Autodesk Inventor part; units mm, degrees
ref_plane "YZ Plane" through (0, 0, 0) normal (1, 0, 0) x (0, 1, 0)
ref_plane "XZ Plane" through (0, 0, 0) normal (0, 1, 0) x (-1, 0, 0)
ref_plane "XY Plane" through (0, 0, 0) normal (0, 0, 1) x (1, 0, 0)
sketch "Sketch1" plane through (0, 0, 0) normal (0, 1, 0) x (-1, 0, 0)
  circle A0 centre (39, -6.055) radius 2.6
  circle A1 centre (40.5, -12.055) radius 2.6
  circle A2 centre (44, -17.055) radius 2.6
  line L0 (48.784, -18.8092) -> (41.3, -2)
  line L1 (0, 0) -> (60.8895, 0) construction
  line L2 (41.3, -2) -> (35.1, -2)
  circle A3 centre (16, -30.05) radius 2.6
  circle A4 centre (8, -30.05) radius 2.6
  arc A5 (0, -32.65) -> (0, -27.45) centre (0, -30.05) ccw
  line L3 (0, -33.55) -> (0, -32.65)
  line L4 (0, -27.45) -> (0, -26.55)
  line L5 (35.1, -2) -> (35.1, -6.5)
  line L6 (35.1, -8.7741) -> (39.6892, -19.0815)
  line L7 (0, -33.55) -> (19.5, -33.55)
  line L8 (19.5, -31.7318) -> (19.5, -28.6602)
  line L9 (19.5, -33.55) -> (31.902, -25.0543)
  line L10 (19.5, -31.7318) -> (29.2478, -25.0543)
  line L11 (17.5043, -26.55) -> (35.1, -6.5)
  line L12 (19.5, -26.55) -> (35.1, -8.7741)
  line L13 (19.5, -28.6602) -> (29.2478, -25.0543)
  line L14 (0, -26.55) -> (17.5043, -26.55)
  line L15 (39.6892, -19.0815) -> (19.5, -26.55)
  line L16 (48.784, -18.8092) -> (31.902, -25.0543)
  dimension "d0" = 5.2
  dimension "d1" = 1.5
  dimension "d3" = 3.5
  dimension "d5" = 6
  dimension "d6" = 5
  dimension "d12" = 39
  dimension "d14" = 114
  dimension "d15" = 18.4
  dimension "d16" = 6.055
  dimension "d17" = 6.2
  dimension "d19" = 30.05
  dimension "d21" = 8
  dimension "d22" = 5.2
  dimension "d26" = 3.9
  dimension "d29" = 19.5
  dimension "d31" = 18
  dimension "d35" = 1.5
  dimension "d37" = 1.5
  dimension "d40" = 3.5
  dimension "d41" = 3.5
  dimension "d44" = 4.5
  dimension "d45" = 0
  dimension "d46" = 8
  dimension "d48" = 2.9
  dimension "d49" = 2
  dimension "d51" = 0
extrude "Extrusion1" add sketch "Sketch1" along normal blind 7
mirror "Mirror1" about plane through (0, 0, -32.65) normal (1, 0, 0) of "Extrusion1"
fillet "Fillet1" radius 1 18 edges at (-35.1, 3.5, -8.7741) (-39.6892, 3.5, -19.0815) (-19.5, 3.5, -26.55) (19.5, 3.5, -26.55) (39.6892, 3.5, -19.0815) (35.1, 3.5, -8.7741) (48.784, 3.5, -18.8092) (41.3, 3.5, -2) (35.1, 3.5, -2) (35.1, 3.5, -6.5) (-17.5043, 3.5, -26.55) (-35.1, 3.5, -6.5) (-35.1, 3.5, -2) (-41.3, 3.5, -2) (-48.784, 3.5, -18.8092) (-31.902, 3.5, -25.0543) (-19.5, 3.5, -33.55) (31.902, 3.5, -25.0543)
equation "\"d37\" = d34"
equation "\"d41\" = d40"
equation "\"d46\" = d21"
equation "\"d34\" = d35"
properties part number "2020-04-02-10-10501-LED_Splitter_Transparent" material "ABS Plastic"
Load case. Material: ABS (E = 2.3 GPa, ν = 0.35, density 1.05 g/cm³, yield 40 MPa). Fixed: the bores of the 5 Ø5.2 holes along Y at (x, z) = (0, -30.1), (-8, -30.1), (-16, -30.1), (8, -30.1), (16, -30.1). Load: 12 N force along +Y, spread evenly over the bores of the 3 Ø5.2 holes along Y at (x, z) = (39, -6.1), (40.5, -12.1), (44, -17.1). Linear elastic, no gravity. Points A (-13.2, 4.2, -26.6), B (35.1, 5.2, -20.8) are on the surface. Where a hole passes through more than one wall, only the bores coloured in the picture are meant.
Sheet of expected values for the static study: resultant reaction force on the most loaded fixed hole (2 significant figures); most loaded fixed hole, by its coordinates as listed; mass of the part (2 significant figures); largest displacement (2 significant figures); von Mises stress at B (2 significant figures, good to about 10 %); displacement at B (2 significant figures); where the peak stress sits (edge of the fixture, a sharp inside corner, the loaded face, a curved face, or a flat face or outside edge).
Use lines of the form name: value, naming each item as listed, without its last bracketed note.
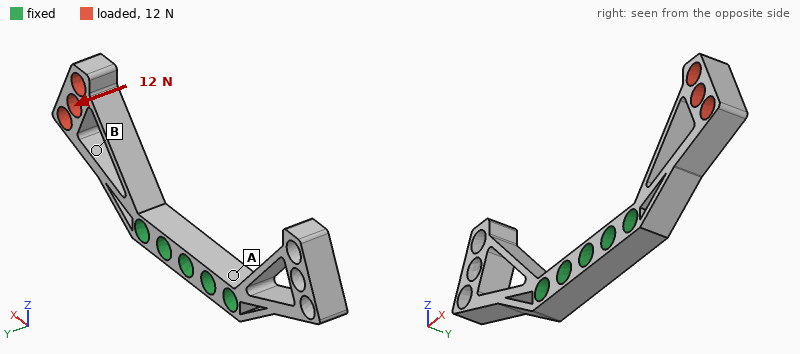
resultant reaction force on the most loaded fixed hole: 12 N
most loaded fixed hole, by its coordinates as listed: (16, -30.1)
mass of the part: 4.3 g
largest displacement: 0.49 mm
von Mises stress at B: 3.2 MPa
displacement at B: 0.16 mm
where the peak stress sits: a curved face
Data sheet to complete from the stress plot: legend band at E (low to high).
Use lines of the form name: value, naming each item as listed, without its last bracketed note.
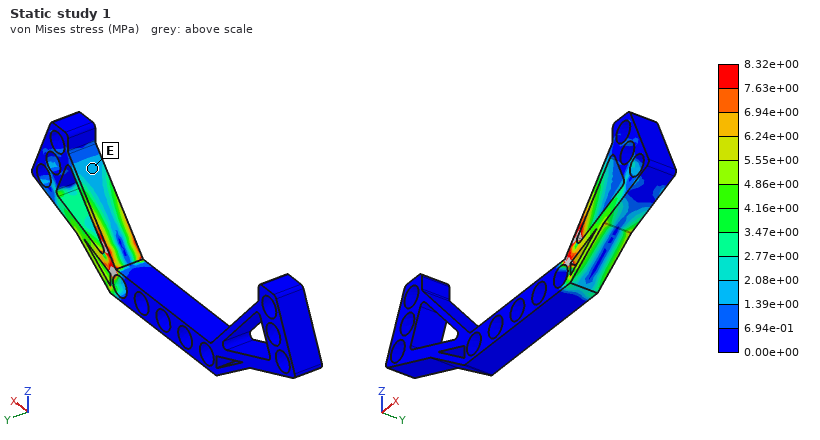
legend band at E: 1.39e+00 to 2.08e+00 MPa
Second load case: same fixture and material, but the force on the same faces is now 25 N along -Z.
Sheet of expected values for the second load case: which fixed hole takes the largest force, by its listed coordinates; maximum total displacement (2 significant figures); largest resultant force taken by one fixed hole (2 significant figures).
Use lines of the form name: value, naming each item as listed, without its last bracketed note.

which fixed hole takes the largest force, by its listed coordinates: (16, -30.1)
maximum total displacement: 1.0 mm
largest resultant force taken by one fixed hole: 27 N
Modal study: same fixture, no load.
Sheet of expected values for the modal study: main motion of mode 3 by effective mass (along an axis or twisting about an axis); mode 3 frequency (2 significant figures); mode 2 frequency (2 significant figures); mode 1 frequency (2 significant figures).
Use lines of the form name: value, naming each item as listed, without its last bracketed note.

main motion of mode 3 by effective mass: along Y
mode 3 frequency: 1000 Hz
mode 2 frequency: 840 Hz
mode 1 frequency: 840 Hz
